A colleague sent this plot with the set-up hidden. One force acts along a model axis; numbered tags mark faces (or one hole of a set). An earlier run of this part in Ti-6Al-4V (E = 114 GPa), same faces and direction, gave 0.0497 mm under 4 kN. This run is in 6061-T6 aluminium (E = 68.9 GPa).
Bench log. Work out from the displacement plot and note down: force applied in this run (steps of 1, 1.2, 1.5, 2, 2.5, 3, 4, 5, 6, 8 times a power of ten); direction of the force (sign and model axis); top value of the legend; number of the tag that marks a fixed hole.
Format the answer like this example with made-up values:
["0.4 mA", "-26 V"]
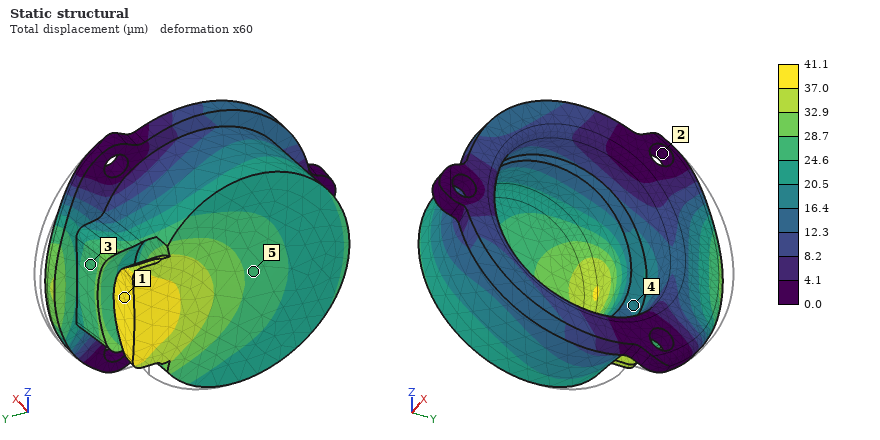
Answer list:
["2 kN", "-Y", "41.1 µm", "2"]
